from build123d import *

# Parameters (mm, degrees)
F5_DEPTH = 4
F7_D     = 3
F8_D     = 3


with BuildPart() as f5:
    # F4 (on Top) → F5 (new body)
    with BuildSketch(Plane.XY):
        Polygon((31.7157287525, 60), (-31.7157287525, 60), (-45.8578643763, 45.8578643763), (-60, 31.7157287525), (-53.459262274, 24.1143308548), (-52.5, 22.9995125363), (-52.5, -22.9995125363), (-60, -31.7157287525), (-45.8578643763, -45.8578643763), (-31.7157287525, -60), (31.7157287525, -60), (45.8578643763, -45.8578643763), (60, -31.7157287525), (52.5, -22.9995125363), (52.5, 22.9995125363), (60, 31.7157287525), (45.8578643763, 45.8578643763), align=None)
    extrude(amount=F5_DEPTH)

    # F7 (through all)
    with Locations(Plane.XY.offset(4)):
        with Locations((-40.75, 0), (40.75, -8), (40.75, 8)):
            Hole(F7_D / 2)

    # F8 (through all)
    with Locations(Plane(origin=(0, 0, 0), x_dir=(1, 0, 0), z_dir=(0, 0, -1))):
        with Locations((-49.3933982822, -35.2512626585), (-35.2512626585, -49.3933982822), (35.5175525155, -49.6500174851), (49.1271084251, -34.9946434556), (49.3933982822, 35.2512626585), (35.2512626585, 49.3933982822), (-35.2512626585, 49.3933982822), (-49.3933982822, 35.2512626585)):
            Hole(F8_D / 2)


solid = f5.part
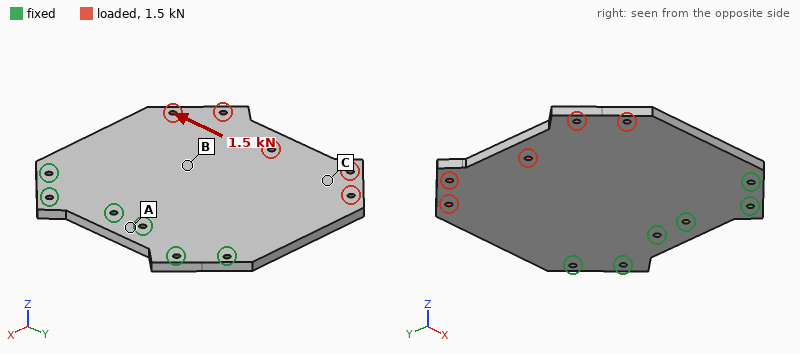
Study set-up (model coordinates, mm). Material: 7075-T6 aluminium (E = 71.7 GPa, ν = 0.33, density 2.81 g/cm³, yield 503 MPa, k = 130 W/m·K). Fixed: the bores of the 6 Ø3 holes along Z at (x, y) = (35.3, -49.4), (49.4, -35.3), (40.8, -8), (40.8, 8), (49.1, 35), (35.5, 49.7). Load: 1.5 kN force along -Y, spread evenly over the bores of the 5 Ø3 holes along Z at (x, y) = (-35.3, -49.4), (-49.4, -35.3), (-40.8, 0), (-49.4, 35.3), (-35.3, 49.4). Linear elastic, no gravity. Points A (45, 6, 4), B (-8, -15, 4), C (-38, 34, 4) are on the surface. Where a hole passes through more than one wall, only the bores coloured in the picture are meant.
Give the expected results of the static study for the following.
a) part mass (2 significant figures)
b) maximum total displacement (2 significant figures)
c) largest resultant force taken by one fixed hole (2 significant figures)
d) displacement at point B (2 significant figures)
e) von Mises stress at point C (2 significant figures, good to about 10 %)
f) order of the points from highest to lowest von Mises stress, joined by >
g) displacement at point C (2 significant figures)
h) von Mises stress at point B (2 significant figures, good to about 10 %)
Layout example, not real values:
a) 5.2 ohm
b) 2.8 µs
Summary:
a) 130 g
b) 23 µm
c) 1.0 kN
d) 10 µm
e) 4.3 MPa
f) B > C > A
g) 19 µm
h) 7.7 MPa
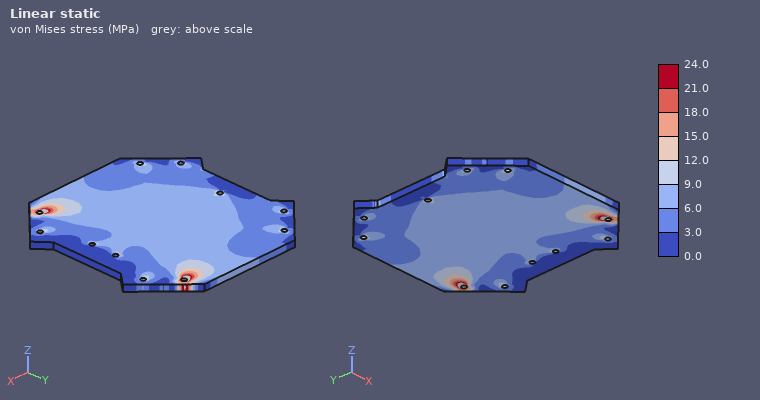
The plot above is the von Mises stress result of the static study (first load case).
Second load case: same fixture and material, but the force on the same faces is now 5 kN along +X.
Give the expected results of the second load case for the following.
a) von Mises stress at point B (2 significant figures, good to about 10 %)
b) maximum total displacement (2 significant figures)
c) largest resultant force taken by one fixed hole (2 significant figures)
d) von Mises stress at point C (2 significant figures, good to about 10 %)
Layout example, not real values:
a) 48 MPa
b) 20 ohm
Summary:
a) 8.6 MPa
b) 17 µm
c) 1.1 kN
d) 14 MPa
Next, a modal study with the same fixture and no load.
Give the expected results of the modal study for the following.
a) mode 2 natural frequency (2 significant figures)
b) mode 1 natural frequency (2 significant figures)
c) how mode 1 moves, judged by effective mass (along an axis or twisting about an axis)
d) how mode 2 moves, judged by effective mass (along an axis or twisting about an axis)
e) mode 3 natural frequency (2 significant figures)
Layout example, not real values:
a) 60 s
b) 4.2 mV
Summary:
a) 910 Hz
b) 400 Hz
c) along Z
d) twisting about X
e) 2100 Hz
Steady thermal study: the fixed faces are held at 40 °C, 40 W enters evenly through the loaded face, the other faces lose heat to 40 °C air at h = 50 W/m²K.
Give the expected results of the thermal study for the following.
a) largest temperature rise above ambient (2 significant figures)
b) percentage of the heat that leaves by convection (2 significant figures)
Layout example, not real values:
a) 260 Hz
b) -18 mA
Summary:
a) 41 K
b) 50 %
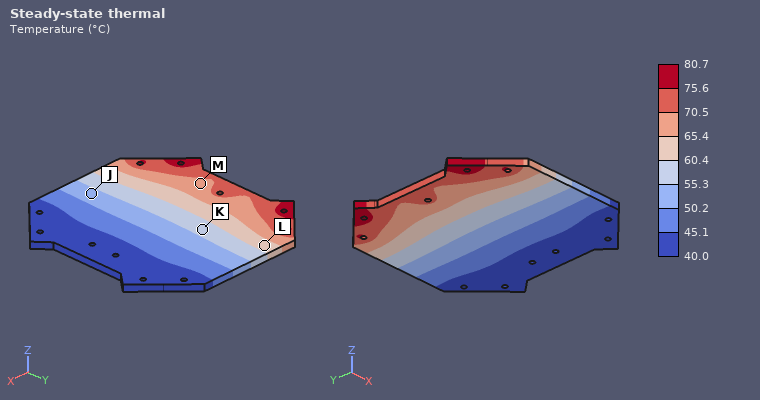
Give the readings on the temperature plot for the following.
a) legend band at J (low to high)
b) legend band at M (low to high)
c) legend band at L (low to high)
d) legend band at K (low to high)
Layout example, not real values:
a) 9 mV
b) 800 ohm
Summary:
a) 50.2 to 55.3 °C
b) 65.4 to 70.5 °C
c) 60.4 to 65.4 °C
d) 55.3 to 60.4 °C
